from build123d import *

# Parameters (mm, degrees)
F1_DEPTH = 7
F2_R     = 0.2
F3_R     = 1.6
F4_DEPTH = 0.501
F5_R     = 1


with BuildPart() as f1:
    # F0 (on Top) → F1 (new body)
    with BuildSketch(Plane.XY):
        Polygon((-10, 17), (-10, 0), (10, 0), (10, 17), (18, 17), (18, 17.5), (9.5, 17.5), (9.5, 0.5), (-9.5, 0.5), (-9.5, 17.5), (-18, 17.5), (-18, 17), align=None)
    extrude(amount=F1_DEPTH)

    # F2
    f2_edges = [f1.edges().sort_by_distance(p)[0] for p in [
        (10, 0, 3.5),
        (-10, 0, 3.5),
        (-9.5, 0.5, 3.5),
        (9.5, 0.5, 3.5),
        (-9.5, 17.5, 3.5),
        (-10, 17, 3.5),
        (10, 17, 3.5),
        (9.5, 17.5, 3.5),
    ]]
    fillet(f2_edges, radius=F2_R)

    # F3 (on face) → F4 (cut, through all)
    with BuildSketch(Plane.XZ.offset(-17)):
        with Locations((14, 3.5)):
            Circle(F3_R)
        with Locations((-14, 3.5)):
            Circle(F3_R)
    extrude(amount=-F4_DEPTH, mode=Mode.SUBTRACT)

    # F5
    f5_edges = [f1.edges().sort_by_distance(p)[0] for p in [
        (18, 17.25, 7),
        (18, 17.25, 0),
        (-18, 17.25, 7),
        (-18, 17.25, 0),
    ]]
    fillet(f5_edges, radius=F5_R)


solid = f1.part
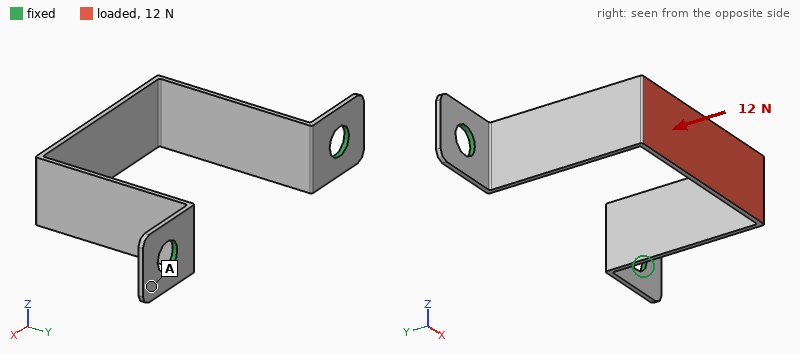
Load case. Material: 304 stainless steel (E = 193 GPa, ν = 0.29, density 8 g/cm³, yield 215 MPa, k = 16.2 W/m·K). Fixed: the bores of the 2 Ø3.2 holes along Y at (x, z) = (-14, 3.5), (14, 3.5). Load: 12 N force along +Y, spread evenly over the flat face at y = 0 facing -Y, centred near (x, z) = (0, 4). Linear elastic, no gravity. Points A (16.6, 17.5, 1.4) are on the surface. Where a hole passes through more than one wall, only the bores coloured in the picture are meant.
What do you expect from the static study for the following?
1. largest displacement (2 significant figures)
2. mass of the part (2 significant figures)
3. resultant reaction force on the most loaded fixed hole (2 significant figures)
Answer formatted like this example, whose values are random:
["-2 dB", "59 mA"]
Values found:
["36 µm", "1.9 g", "6.1 N"]
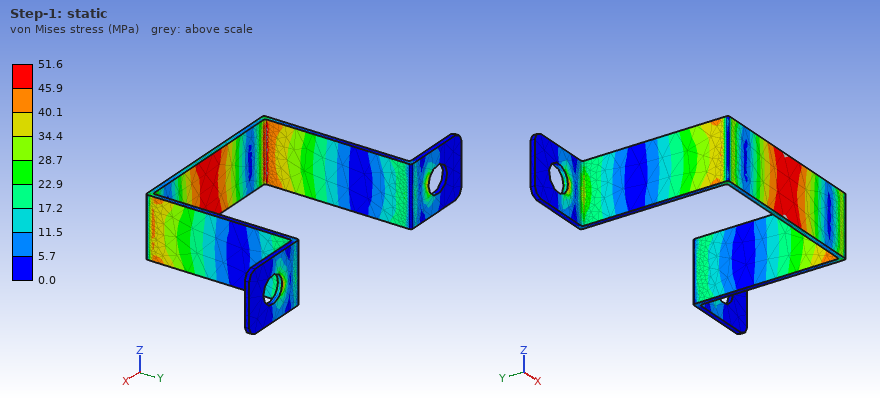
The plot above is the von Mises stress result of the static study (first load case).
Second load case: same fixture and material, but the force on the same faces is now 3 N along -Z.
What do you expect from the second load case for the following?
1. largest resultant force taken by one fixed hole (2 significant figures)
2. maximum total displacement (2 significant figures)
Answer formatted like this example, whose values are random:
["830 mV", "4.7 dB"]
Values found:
["1.5 N", "36 µm"]
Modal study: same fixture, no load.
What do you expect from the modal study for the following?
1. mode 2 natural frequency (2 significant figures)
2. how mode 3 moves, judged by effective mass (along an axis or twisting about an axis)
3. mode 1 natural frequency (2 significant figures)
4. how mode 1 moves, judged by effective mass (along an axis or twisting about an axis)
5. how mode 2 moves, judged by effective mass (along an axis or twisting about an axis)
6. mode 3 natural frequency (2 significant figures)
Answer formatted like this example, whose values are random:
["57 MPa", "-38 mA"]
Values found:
["1600 Hz", "twisting about Y", "1100 Hz", "along X", "along Z", "2400 Hz"]
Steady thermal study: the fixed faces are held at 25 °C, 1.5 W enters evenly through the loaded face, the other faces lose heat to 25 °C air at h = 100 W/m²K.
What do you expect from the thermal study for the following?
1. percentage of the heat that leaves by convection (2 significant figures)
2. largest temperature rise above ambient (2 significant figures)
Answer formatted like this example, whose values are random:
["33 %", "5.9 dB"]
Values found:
["97 %", "62 K"]
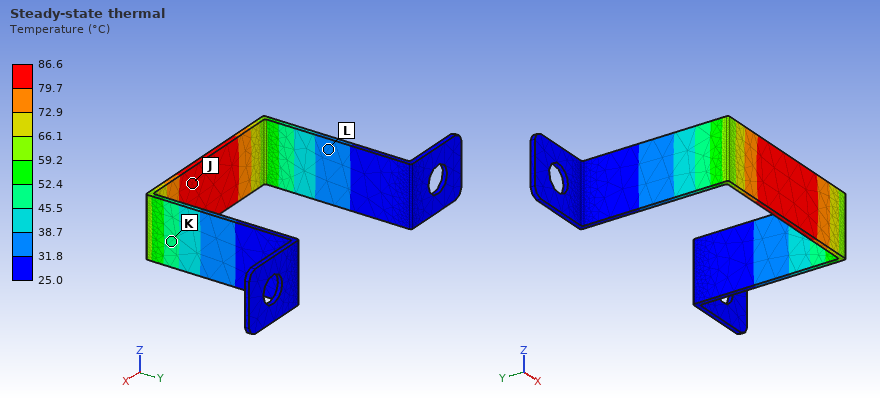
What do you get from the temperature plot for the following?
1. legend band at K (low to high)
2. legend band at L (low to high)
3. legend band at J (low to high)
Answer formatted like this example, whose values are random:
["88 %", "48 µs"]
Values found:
["45.5 to 52.4 °C", "31.8 to 38.7 °C", "79.7 to 86.6 °C"]
